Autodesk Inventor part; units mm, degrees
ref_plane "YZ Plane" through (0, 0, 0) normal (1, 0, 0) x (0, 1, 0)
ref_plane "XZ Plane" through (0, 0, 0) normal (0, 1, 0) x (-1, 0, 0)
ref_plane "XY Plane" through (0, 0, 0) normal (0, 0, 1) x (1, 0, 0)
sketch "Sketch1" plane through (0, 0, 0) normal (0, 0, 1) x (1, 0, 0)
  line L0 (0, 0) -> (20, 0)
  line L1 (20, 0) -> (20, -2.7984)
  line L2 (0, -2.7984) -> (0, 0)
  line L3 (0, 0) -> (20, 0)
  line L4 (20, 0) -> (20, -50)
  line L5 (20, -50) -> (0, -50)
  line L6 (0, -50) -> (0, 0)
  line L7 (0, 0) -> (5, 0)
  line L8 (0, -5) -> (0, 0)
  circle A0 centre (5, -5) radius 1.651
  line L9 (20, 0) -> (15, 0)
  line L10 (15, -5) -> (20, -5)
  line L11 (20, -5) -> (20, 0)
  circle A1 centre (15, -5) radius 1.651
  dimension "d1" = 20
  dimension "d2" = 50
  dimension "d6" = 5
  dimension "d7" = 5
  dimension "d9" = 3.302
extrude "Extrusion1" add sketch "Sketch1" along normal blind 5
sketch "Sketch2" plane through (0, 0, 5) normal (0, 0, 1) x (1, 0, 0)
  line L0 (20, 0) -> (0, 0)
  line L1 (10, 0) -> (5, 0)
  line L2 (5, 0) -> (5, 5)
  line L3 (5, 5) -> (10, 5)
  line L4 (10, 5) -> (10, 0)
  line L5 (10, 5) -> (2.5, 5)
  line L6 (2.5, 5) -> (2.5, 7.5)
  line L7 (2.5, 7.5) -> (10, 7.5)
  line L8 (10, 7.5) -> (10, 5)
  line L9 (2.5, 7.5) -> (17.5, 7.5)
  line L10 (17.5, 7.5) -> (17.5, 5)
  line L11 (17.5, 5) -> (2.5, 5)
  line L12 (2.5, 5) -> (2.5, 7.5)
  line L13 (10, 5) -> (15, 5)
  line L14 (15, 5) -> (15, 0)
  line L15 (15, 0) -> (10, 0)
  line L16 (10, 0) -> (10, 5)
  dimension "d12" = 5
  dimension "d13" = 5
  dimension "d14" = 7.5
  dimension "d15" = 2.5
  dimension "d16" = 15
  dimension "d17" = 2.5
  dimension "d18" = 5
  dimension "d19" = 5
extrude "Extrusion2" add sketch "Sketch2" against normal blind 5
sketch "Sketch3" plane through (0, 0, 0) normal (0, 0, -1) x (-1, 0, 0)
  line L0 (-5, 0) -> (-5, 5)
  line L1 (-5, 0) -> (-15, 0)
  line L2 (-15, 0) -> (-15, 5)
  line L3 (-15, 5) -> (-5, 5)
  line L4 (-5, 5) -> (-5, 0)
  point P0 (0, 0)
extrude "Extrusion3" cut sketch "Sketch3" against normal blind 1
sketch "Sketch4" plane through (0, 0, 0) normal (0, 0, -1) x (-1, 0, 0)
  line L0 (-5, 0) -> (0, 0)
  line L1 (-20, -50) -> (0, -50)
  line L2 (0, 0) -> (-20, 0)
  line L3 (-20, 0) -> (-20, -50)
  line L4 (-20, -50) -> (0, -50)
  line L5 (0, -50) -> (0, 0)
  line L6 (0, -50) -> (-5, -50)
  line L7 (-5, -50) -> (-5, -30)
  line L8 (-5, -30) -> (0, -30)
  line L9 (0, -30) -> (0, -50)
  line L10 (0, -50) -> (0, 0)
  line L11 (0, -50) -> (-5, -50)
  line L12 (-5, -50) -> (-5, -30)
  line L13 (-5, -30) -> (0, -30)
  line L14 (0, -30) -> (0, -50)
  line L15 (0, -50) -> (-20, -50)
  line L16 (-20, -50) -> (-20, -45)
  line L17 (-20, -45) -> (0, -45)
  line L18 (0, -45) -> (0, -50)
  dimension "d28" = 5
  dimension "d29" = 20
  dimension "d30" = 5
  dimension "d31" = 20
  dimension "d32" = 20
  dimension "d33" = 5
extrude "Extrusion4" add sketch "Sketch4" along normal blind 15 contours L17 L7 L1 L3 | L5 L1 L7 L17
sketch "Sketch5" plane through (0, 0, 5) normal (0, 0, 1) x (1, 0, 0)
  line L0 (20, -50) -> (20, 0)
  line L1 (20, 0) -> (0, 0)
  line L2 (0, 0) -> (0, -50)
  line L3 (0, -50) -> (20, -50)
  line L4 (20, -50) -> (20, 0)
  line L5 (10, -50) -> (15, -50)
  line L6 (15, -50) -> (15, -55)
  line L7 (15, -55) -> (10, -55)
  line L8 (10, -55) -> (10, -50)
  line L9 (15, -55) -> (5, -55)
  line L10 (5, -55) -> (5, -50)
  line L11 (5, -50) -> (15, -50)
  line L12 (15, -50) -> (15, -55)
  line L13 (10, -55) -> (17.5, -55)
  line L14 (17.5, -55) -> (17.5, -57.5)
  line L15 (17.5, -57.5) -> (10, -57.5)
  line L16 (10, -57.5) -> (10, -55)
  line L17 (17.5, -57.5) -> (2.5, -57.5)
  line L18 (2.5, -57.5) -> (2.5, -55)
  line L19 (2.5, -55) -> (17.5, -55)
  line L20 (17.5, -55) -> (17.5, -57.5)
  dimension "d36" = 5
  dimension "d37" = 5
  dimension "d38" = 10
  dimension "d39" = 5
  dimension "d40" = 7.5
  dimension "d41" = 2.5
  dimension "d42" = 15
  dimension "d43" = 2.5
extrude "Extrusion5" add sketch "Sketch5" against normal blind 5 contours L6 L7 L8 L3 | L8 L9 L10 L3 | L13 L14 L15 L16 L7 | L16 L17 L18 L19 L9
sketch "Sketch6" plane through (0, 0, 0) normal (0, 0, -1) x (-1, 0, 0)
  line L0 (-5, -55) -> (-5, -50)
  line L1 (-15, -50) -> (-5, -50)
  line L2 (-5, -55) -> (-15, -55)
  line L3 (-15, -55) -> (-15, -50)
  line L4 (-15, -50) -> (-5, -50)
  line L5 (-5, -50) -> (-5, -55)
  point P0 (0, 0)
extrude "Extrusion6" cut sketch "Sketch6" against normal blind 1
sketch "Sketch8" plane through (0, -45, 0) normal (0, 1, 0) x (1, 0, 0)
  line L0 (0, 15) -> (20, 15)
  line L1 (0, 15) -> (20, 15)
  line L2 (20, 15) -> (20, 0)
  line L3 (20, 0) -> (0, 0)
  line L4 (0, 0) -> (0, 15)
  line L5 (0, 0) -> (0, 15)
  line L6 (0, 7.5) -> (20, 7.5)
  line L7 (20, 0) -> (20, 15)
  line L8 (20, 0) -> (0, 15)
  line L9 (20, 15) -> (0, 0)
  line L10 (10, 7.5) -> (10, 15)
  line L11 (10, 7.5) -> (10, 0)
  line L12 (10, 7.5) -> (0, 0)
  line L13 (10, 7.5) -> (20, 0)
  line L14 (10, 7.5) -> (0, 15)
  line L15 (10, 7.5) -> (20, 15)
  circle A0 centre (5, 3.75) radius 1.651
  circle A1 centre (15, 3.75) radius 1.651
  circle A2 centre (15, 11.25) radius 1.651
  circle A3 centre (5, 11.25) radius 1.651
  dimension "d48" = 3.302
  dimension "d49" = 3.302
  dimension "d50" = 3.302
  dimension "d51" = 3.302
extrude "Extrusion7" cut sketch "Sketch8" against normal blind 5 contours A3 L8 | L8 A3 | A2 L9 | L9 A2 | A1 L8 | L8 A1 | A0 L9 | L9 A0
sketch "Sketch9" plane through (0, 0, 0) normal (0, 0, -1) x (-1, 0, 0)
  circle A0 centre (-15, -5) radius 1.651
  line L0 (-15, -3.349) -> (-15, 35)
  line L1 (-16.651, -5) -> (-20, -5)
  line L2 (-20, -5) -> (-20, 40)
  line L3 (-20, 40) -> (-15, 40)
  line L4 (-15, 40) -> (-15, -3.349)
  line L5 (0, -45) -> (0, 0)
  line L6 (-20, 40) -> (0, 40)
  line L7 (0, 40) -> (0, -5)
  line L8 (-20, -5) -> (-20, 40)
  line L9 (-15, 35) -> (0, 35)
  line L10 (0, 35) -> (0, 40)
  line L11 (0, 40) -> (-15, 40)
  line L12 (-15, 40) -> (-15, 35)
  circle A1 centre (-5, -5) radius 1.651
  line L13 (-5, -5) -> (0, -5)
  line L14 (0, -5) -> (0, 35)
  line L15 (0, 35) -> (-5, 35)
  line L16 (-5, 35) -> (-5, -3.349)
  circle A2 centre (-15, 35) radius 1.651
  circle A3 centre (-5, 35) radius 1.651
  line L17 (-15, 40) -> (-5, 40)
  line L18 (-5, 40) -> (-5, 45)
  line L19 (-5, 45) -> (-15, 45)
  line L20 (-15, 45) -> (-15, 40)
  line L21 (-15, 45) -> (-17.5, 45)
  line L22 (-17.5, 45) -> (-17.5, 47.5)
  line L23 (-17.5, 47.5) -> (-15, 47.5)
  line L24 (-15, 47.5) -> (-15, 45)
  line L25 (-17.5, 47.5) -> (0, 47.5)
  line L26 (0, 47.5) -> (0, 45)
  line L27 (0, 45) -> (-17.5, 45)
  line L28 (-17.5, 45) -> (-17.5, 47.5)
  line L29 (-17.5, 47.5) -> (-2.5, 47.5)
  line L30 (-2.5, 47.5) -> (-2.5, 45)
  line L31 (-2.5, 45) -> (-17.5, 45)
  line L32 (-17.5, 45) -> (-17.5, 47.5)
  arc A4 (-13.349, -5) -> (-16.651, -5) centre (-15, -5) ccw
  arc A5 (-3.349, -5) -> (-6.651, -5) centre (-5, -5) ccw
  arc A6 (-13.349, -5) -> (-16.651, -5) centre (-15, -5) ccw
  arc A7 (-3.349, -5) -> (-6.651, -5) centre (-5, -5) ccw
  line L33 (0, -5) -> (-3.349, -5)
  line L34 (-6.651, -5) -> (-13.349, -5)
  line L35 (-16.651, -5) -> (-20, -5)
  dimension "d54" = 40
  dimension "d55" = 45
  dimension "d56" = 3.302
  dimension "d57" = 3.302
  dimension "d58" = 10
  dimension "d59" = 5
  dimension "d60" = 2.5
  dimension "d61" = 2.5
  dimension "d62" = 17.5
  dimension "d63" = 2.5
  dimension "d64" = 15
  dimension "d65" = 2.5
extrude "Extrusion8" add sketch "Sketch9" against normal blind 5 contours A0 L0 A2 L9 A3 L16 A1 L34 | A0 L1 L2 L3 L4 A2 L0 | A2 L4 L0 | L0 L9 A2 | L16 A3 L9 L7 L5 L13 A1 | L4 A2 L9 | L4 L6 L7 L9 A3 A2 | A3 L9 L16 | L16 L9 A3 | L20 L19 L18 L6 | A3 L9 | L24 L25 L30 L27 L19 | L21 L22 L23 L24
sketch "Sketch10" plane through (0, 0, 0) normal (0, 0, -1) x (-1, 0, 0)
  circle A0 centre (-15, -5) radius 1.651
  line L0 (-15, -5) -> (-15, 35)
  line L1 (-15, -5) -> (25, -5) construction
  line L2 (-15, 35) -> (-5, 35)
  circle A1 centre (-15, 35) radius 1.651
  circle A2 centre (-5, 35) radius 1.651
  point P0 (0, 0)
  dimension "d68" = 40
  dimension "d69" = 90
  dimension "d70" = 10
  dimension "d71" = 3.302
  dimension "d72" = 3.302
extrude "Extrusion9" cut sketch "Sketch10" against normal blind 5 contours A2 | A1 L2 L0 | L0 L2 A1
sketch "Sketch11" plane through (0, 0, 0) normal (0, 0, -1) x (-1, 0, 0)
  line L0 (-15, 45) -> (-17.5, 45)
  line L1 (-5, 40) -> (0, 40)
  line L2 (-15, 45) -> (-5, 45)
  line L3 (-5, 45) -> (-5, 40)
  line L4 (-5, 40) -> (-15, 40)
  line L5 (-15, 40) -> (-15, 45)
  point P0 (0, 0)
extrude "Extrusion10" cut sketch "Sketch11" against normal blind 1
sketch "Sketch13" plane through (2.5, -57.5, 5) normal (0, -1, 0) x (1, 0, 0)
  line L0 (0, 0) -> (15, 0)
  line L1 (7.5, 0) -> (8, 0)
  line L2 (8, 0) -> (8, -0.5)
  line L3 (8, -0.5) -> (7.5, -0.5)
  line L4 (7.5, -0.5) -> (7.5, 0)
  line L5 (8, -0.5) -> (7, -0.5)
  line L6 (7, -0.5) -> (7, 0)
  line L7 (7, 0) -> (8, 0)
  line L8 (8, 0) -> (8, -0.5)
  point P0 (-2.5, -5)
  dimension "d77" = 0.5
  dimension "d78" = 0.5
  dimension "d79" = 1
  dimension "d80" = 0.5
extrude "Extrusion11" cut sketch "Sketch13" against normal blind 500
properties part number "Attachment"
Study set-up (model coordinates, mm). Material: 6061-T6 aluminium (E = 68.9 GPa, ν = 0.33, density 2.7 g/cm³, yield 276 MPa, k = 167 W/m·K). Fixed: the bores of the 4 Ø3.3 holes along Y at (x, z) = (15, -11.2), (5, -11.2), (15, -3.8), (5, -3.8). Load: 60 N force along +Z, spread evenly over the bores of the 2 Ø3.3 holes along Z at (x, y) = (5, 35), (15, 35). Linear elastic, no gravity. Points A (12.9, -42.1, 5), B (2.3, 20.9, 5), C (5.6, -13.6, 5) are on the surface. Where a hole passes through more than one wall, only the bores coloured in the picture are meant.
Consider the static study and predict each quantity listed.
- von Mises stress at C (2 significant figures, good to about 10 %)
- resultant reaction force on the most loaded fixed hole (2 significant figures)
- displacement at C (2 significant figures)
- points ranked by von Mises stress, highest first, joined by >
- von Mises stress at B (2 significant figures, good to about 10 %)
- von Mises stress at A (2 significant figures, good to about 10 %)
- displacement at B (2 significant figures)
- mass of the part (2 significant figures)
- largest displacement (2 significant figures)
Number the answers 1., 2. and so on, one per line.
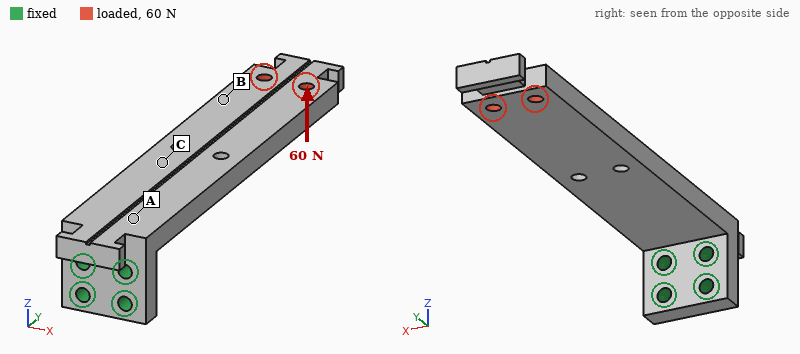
1. 35 MPa
2. 94 N
3. 0.22 mm
4. A > C > B
5. 10 MPa
6. 53 MPa
7. 0.69 mm
8. 29 g
9. 1.1 mm
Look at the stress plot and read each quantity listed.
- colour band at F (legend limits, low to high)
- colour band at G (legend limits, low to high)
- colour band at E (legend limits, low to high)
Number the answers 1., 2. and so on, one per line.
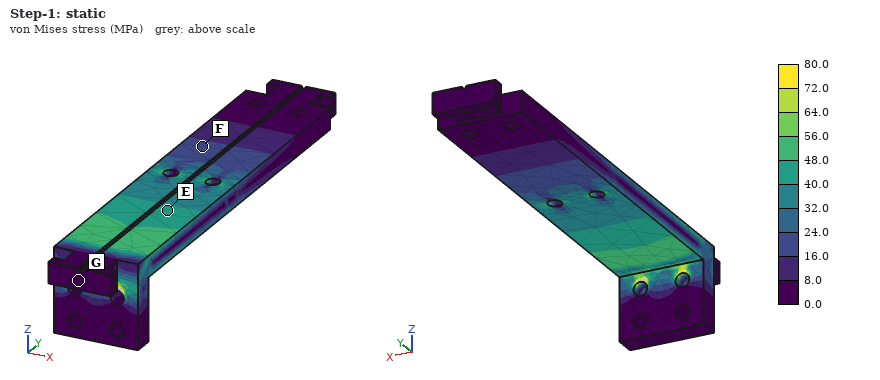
1. 16.0 to 24.0 MPa
2. 0.0 to 8.0 MPa
3. 40.0 to 48.0 MPa
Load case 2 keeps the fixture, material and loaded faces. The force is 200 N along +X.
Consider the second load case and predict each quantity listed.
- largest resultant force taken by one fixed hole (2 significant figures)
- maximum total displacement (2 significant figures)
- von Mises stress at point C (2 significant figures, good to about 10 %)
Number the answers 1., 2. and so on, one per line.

1. 1.2 kN
2. 0.35 mm
3. 13 MPa
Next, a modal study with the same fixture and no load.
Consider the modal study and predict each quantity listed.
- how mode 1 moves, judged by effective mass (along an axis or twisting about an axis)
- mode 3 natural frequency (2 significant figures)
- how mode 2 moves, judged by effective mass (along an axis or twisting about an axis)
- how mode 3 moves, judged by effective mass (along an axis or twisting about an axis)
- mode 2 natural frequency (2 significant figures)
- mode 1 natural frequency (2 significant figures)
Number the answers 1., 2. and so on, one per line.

1. along Z
2. 2700 Hz
3. along X
4. along Z
5. 1400 Hz
6. 450 Hz
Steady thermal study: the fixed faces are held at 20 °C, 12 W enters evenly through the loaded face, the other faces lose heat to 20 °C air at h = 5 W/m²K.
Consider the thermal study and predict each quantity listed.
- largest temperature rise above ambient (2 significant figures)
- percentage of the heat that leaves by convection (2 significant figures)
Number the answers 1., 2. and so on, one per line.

1. 62 K
2. 7.2 %
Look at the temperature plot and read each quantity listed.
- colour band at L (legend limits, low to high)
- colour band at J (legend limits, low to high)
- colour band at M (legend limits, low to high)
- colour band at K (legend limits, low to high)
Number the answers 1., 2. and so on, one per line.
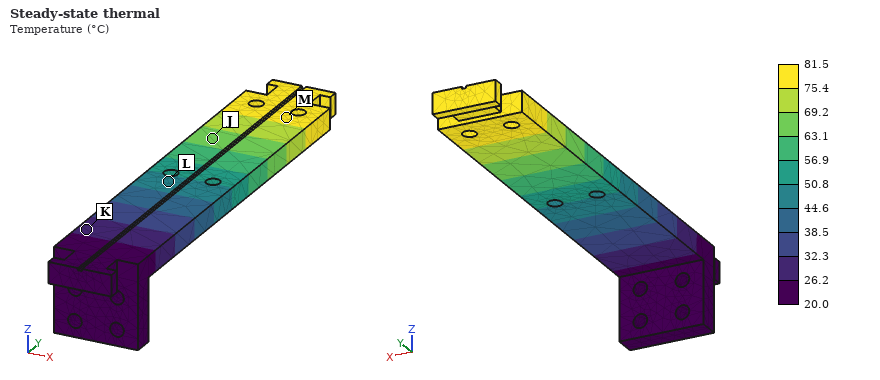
1. 44.6 to 50.8 °C
2. 63.1 to 69.2 °C
3. 75.4 to 81.5 °C
4. 26.2 to 32.3 °C
